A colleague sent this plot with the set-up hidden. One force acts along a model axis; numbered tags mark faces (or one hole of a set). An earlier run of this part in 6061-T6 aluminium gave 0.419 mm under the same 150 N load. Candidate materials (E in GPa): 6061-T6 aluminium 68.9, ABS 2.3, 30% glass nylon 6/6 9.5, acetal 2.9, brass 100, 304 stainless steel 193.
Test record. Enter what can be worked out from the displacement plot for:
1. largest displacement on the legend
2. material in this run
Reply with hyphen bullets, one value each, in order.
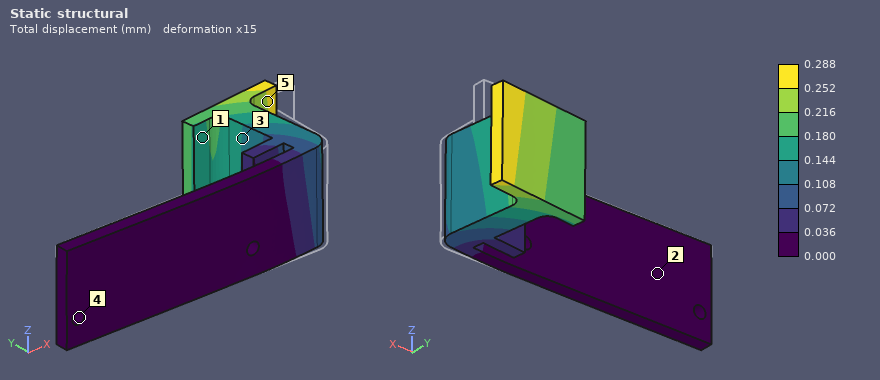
- 0.288 mm
- brass
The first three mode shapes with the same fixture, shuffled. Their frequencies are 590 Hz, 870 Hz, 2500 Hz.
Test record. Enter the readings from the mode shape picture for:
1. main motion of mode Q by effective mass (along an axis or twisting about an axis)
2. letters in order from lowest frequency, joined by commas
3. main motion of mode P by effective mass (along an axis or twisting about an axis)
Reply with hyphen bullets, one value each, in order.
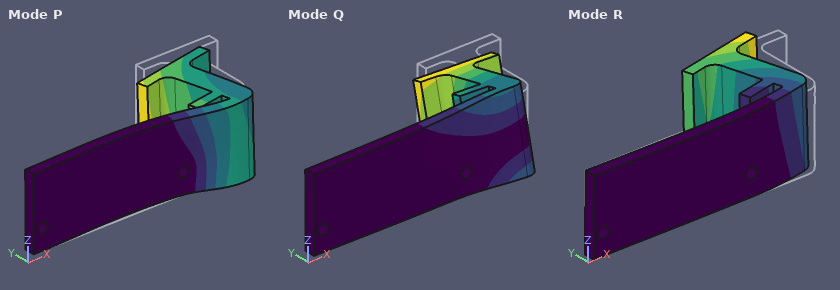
- along Z
- R, Q, P
- along Y
